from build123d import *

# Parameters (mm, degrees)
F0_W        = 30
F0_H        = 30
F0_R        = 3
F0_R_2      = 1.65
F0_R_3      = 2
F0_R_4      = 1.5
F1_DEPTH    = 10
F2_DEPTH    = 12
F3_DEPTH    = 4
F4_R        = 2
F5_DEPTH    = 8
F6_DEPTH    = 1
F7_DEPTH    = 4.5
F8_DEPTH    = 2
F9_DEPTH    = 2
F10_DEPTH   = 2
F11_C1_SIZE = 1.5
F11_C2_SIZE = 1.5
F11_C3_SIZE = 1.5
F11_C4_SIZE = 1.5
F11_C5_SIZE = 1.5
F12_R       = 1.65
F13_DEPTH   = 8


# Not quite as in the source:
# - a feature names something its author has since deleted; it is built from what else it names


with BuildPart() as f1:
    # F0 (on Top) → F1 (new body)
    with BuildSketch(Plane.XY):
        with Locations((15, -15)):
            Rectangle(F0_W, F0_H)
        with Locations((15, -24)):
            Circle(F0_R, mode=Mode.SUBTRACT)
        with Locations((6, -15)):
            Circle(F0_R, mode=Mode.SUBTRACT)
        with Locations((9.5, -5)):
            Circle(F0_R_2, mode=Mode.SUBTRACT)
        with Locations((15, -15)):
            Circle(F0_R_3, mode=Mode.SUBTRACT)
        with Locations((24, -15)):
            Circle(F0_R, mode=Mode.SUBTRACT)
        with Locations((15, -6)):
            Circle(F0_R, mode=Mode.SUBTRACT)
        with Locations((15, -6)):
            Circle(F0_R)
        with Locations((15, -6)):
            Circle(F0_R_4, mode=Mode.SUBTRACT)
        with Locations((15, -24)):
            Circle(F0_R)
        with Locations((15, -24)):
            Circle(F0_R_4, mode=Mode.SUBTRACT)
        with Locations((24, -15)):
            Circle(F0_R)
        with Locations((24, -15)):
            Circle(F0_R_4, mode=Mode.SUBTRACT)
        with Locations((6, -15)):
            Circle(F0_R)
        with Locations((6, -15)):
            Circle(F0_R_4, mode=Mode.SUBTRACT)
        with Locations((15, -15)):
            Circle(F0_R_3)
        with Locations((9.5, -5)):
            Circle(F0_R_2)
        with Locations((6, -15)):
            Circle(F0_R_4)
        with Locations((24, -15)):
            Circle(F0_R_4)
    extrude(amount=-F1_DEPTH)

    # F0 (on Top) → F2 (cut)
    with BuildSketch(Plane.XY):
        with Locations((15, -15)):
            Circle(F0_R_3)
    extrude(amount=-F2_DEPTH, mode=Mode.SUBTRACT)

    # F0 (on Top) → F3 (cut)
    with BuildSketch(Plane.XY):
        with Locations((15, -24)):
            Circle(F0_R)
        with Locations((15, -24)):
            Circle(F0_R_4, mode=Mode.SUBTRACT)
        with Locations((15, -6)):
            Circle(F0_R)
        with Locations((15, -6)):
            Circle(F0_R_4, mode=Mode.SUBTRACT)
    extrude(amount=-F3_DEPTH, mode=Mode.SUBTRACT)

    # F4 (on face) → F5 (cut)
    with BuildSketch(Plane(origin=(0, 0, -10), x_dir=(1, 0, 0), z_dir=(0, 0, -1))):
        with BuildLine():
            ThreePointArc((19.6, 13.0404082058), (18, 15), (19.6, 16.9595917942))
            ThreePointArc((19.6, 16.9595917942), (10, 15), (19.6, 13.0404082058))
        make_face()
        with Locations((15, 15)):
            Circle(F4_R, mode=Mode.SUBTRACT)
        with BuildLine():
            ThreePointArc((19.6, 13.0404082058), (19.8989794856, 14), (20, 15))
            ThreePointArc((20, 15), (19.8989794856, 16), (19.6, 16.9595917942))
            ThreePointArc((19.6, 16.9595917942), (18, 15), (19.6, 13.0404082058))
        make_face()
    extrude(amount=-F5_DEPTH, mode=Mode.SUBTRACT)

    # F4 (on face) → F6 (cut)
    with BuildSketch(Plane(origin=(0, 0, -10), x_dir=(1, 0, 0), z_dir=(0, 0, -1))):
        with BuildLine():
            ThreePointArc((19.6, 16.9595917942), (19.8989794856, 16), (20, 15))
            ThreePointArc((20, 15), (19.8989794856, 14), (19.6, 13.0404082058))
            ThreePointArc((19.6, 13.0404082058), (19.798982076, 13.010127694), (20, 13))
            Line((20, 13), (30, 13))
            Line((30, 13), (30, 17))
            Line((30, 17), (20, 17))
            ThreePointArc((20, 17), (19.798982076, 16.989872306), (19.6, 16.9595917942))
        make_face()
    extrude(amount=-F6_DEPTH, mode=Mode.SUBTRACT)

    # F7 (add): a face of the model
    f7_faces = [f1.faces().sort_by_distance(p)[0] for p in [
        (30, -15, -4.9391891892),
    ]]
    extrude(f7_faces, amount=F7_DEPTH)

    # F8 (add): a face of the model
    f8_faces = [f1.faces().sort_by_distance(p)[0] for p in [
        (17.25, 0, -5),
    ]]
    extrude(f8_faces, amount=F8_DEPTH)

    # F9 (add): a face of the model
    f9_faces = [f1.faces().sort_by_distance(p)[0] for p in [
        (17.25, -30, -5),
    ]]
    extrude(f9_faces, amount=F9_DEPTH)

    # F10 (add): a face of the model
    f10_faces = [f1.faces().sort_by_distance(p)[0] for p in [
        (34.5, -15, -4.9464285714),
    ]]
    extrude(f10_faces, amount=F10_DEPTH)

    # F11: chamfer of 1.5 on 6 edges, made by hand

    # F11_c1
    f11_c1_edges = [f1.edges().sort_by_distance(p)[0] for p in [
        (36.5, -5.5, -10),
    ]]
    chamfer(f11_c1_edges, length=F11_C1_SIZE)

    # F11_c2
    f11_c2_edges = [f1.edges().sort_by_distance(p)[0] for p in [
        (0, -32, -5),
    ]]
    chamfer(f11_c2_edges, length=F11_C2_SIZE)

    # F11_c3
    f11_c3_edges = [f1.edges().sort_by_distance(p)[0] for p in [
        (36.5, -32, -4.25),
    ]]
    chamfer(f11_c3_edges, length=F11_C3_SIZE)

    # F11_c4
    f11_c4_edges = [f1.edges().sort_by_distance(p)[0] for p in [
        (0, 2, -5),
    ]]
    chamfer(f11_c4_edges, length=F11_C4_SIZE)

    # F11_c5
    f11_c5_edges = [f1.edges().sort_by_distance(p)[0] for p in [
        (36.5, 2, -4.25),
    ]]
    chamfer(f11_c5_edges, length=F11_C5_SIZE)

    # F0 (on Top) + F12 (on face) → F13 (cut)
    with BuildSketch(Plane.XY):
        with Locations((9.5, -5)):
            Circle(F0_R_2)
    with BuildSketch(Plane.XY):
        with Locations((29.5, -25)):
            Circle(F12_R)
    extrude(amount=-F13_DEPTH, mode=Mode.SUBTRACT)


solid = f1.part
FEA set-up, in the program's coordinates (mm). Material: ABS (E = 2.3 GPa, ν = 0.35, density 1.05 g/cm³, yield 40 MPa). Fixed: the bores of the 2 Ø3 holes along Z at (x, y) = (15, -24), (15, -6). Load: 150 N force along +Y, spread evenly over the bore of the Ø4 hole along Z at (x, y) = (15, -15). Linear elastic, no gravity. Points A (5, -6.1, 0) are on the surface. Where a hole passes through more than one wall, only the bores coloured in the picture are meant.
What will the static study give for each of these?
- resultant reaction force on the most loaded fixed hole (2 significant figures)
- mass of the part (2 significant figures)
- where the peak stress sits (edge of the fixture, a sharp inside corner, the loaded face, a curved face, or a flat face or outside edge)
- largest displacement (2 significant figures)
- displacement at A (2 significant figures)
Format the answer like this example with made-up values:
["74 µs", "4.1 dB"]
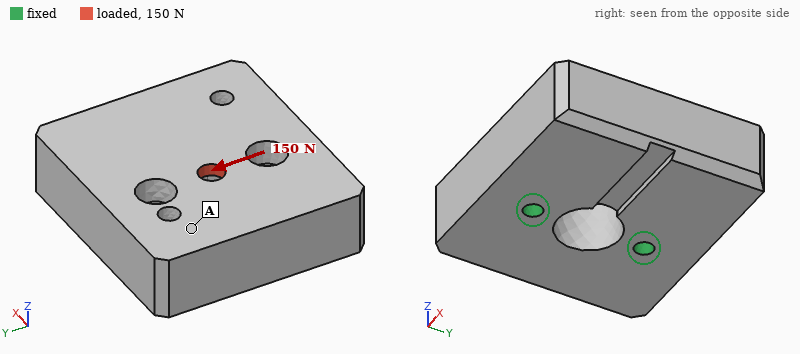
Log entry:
["83 N", "12 g", "the loaded face", "23 µm", "8.5 µm"]
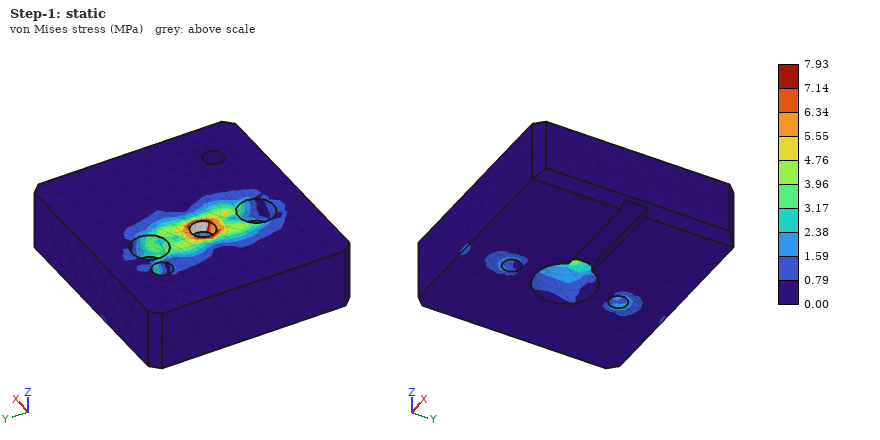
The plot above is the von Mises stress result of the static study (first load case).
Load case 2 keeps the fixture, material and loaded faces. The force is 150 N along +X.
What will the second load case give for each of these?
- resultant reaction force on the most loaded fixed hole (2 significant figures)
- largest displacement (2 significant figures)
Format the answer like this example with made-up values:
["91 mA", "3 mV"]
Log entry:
["75 N", "53 µm"]
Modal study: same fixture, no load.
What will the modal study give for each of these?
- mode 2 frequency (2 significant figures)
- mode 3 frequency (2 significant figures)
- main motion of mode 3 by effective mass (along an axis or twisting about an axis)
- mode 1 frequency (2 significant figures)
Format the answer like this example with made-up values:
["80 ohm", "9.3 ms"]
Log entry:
["5000 Hz", "5600 Hz", "along Y", "2400 Hz"]
